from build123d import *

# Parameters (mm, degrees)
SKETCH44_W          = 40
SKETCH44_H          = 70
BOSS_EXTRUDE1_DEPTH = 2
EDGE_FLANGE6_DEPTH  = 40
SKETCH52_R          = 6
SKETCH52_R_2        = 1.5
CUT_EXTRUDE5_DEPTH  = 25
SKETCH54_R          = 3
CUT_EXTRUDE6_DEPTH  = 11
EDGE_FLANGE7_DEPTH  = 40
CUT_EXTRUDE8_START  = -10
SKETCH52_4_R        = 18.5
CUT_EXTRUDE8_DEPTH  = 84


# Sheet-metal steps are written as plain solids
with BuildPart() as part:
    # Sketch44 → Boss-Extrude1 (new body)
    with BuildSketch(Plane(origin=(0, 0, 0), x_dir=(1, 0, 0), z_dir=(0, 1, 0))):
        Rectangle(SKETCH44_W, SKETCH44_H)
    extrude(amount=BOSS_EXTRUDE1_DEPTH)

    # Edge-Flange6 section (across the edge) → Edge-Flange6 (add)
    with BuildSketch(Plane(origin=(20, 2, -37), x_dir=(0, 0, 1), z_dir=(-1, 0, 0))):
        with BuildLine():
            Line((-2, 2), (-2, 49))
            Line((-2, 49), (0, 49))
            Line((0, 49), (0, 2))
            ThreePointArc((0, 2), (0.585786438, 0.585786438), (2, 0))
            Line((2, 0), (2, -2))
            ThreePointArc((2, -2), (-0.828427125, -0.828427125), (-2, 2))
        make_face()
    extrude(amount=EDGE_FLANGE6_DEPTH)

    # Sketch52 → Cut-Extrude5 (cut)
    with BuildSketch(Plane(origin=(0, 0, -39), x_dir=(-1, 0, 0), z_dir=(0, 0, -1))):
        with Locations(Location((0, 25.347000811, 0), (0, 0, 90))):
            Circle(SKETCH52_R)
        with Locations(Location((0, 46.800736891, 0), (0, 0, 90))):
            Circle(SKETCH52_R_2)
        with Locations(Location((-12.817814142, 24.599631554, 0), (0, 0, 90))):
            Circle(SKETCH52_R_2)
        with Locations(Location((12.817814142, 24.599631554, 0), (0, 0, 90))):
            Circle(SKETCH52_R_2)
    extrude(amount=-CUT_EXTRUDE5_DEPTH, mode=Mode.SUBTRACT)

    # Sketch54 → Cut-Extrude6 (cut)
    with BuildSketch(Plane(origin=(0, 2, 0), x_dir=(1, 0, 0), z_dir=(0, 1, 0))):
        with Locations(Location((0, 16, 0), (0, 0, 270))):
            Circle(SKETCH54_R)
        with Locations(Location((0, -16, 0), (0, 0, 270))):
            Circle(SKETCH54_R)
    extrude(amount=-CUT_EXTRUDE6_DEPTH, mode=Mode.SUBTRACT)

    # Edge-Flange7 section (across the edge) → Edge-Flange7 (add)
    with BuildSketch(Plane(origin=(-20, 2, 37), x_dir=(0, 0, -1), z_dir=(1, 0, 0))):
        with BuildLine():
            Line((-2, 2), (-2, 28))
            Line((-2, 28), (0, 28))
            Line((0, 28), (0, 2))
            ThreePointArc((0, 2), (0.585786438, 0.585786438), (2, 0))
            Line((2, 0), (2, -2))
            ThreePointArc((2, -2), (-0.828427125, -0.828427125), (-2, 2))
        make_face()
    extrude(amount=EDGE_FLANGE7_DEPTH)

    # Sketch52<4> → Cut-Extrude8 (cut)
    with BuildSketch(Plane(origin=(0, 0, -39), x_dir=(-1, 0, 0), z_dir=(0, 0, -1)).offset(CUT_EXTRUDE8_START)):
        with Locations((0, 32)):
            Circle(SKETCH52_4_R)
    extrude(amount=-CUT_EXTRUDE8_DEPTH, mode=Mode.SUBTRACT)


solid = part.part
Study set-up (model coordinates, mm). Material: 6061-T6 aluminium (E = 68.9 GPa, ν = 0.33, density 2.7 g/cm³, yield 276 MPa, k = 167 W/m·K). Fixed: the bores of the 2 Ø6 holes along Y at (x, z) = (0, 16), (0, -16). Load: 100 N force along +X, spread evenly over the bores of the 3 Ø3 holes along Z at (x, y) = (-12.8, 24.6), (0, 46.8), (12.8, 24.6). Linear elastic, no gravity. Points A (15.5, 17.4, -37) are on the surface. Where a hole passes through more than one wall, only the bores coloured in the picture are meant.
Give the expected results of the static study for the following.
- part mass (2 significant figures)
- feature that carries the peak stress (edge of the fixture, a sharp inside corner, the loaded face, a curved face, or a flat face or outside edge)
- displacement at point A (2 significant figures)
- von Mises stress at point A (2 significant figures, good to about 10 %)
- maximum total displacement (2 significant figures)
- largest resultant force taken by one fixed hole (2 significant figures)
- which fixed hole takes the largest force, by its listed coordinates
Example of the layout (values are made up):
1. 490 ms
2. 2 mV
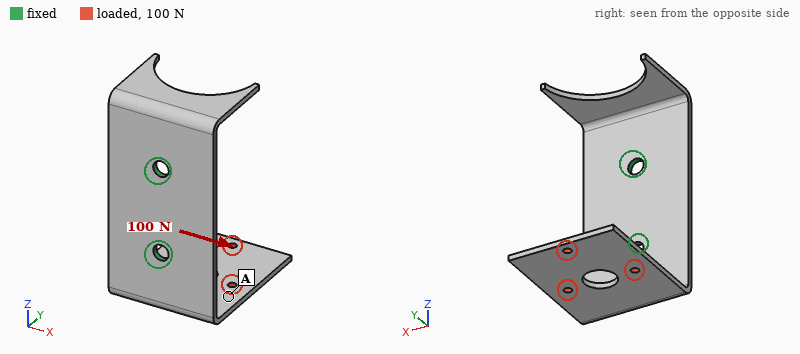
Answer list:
1. 29 g
2. a flat face or outside edge
3. 0.44 mm
4. 18 MPa
5. 1.0 mm
6. 150 N
7. (0, -16)
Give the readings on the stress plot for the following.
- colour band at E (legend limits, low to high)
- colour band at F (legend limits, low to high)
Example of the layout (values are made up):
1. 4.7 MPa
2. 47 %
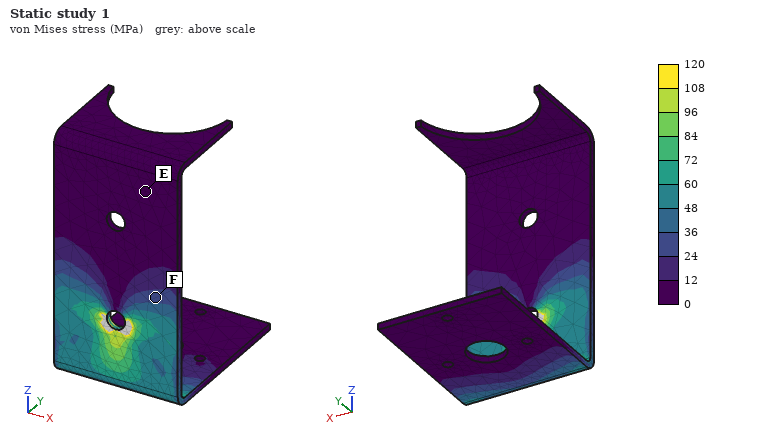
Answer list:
1. 0 to 12 MPa
2. 24 to 36 MPa
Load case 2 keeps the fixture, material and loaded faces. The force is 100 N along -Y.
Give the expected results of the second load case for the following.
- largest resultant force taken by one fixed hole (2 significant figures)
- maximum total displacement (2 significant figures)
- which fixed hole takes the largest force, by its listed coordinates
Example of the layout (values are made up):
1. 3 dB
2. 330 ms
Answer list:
1. 110 N
2. 0.65 mm
3. (0, -16)
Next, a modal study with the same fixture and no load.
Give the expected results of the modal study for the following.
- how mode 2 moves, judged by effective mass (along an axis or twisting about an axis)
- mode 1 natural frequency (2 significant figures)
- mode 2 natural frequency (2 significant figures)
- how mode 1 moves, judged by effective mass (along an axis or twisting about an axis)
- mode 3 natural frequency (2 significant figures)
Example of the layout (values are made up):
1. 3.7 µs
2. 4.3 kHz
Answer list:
1. along X
2. 400 Hz
3. 630 Hz
4. along Z
5. 1400 Hz
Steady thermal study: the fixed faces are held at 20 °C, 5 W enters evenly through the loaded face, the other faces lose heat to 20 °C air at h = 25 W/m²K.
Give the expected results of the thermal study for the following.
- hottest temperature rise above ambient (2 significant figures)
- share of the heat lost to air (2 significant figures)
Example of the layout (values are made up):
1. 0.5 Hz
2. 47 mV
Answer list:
1. 18 K
2. 31 %
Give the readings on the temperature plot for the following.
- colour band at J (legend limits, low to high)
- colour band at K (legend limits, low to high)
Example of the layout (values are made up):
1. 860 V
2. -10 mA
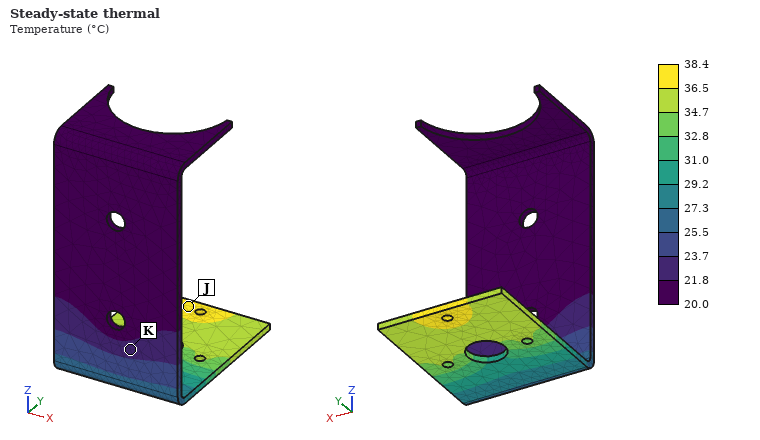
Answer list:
1. 36.5 to 38.4 °C
2. 21.8 to 23.7 °C
